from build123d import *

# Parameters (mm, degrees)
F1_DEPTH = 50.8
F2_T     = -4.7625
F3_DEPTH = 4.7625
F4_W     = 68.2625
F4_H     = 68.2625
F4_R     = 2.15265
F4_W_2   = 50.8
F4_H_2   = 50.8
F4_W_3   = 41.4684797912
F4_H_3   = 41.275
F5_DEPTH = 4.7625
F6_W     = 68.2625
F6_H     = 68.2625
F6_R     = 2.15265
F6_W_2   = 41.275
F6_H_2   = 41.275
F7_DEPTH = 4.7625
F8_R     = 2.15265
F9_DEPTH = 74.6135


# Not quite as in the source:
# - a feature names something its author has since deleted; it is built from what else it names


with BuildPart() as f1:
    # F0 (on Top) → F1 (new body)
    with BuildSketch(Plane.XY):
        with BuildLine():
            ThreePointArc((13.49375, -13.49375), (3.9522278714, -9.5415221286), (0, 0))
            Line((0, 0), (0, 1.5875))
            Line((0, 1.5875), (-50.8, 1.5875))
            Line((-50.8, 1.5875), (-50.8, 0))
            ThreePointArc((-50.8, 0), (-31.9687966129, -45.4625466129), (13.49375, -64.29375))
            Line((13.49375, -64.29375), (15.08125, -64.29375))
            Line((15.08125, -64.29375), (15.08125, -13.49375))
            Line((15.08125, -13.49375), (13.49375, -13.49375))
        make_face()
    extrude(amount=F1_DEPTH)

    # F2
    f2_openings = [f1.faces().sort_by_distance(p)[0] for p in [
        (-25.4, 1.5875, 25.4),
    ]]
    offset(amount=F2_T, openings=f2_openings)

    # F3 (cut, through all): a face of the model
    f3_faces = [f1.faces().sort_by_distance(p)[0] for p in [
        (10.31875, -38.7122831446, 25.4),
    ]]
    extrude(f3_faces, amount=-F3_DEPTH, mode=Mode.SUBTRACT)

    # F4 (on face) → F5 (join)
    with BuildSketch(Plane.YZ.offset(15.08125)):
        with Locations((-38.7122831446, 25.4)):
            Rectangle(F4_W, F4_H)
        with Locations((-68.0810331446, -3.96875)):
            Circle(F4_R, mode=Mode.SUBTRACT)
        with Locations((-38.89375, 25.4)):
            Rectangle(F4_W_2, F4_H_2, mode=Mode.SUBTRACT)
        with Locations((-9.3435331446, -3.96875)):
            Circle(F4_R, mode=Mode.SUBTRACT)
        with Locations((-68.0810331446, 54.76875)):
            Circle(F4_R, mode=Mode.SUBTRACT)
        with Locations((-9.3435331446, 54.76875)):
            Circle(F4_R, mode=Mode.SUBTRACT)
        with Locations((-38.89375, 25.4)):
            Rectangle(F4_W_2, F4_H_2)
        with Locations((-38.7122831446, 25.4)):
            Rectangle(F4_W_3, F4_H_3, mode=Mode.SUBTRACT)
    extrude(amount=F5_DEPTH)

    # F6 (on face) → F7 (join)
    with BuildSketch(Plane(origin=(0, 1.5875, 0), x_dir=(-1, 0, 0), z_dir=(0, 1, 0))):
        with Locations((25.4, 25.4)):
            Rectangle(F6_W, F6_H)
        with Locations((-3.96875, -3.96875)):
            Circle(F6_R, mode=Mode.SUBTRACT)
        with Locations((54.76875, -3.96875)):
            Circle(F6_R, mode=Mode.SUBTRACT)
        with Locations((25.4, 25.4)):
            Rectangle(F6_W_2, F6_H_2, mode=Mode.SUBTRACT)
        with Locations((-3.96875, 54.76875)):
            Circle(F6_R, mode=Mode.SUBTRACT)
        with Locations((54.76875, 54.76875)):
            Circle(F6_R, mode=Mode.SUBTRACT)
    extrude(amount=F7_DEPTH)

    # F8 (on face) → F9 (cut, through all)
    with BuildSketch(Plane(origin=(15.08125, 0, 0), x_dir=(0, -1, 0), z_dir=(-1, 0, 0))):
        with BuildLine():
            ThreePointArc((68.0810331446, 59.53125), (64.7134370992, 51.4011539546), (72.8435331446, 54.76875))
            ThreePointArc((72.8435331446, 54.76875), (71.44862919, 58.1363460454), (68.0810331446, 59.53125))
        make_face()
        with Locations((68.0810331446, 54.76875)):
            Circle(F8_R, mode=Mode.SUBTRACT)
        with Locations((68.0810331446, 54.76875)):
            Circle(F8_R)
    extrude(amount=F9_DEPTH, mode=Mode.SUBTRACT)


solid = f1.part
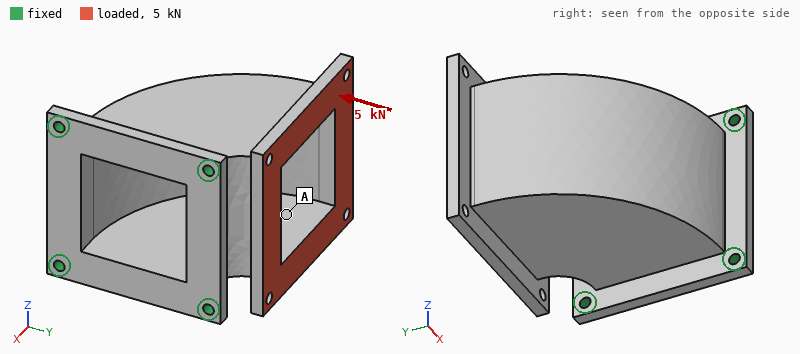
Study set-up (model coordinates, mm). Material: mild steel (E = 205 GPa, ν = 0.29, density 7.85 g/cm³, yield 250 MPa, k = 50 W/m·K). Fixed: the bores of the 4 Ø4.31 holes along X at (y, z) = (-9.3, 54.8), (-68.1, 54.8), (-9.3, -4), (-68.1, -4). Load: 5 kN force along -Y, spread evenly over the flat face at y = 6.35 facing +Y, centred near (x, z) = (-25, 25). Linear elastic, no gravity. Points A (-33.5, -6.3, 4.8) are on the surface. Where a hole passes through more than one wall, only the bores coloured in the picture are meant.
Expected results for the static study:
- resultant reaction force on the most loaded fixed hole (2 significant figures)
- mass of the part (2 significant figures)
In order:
2.5 kN
660 g
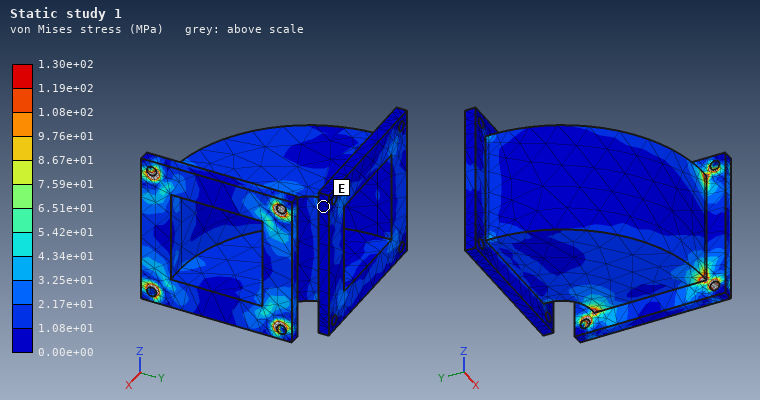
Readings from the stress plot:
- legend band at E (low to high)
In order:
0.00e+00 to 1.08e+01 MPa
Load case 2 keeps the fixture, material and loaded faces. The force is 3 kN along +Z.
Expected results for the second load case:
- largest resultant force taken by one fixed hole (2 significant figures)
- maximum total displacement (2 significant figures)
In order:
2.2 kN
60 µm
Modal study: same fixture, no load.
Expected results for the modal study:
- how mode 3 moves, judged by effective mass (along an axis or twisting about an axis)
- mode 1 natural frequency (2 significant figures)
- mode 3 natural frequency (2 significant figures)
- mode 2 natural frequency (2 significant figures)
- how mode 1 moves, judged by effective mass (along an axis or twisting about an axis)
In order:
along X
2400 Hz
5400 Hz
2600 Hz
along Z
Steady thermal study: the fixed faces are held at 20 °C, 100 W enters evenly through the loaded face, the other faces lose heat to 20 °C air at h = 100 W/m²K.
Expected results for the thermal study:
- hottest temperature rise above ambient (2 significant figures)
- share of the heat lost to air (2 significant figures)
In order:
68 K
87 %
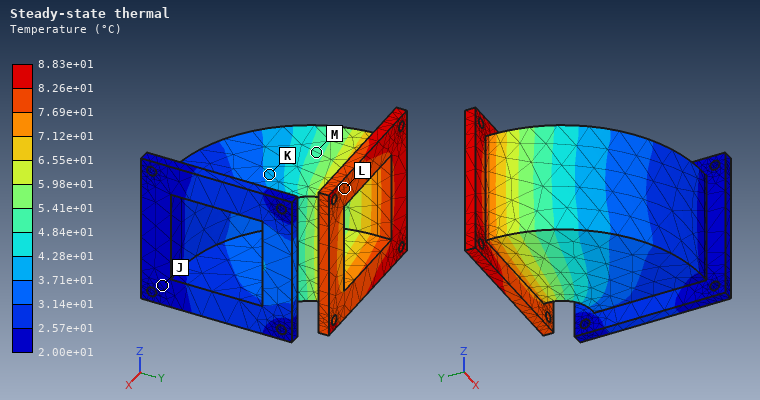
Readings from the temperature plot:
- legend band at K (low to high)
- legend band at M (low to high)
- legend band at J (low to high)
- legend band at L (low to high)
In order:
3.71e+01 to 4.28e+01 °C
4.84e+01 to 5.41e+01 °C
2.00e+01 to 2.57e+01 °C
7.69e+01 to 8.26e+01 °C
